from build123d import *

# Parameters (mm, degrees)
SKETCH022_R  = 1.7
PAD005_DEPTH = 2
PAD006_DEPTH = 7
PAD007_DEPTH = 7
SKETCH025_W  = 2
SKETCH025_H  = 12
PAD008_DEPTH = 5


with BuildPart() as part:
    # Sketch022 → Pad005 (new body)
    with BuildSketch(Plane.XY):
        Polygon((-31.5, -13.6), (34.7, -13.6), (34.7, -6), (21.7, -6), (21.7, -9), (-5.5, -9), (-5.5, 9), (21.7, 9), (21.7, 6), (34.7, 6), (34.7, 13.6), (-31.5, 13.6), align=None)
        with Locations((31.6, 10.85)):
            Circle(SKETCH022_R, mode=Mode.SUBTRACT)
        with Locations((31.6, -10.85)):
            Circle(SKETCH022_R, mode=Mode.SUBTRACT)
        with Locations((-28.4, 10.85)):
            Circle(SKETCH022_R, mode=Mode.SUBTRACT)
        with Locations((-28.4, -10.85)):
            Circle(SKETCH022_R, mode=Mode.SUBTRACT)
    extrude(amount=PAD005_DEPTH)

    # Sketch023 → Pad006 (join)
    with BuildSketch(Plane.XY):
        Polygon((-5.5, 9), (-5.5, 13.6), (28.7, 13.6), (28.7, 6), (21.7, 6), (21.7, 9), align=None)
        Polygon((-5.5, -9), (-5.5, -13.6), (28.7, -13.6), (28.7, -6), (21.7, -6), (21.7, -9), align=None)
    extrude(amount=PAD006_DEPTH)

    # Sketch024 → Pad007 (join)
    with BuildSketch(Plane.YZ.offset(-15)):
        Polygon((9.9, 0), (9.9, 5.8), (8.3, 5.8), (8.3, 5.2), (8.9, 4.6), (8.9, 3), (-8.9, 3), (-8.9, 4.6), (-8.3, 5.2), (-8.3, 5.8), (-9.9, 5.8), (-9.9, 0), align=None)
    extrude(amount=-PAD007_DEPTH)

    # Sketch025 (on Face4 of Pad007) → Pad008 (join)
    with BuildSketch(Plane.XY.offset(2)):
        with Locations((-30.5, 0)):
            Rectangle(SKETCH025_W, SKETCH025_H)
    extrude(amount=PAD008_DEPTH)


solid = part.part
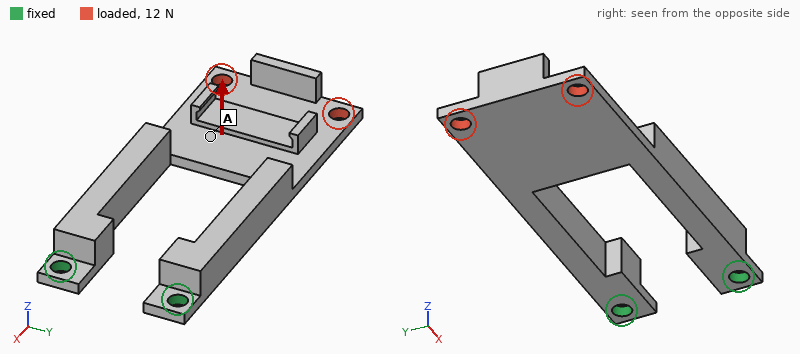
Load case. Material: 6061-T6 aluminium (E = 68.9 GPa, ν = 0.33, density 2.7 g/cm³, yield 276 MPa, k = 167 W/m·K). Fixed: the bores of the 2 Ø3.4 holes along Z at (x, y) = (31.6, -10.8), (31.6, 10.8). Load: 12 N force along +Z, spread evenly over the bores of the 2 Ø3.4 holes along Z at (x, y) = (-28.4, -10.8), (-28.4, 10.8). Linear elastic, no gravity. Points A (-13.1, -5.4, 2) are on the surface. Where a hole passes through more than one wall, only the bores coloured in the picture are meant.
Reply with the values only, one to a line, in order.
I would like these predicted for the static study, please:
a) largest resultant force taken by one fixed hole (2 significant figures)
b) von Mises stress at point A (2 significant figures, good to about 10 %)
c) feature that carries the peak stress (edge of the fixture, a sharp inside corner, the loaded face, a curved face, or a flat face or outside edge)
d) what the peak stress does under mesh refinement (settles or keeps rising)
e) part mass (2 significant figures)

6.0 N
9.0 MPa
edge of the fixture
keeps rising
12 g
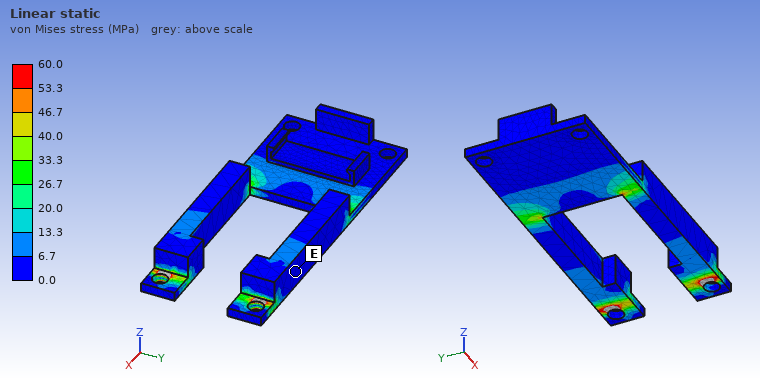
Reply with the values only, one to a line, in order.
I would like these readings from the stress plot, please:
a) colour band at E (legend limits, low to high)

0.0 to 6.7 MPa
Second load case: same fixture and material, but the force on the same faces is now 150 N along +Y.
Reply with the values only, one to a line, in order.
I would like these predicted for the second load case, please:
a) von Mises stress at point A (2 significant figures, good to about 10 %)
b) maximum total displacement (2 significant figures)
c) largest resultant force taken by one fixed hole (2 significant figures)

15 MPa
0.20 mm
240 N
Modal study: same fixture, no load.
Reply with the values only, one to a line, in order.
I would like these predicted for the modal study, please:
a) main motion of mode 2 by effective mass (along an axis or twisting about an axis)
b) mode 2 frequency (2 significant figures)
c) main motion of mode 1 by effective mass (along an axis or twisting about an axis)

along Y
1900 Hz
along Z
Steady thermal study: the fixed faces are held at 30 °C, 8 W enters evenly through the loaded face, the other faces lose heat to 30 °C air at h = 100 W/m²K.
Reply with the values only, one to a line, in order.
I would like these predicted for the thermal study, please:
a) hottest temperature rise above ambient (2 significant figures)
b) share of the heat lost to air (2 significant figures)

34 K
65 %
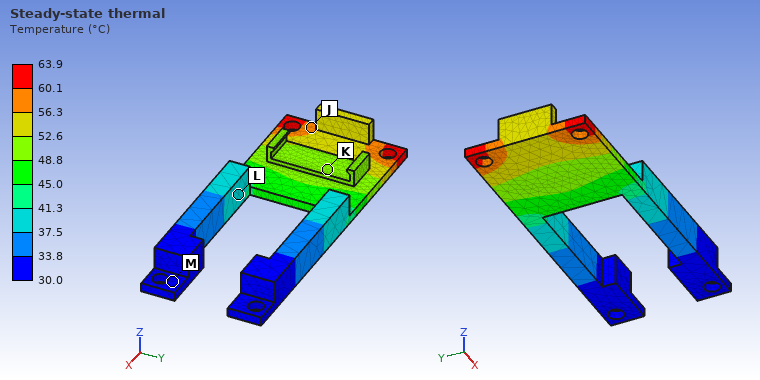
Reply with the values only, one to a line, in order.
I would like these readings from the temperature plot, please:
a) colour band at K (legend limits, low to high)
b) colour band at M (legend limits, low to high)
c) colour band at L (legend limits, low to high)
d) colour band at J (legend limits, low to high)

48.8 to 52.6 °C
30.0 to 33.8 °C
37.5 to 41.3 °C
56.3 to 60.1 °C
